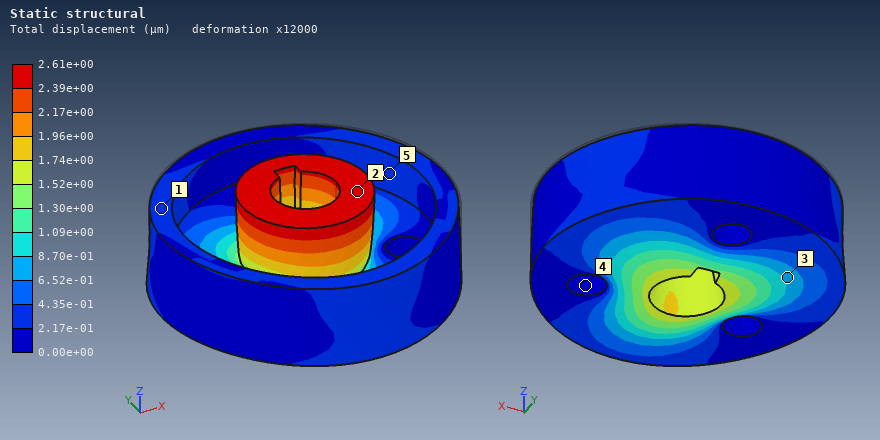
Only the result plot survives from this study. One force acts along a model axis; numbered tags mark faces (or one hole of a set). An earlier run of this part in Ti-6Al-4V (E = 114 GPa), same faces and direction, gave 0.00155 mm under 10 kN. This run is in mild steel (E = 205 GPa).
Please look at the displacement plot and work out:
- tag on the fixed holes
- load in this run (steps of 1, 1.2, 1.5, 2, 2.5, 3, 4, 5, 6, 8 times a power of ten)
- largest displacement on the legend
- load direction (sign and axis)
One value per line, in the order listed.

4
30 kN
2.61e+00 µm
-Z
